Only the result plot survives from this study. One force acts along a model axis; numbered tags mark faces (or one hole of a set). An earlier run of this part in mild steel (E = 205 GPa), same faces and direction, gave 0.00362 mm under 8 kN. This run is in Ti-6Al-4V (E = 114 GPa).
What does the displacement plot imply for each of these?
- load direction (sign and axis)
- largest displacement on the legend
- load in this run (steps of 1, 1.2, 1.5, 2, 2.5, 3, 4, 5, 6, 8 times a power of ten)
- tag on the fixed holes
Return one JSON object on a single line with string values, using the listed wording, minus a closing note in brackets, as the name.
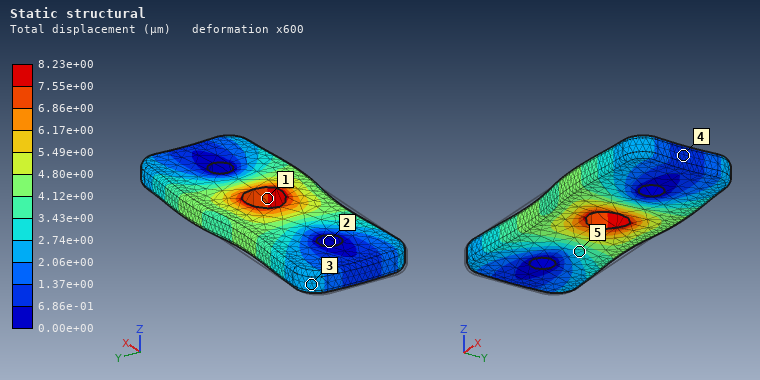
{"load direction": "+X", "largest displacement on the legend": "8.23e+00 µm", "load in this run": "10 kN", "tag on the fixed holes": "2"}
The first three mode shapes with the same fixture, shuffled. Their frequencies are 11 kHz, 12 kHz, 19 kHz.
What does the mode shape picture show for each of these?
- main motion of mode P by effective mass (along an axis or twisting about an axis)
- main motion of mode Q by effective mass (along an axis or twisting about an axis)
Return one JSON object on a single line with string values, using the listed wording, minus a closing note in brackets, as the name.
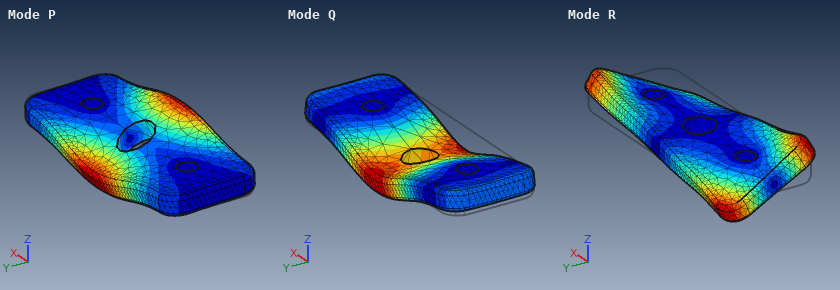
{"main motion of mode P by effective mass": "twisting about X", "main motion of mode Q by effective mass": "along Z"}
